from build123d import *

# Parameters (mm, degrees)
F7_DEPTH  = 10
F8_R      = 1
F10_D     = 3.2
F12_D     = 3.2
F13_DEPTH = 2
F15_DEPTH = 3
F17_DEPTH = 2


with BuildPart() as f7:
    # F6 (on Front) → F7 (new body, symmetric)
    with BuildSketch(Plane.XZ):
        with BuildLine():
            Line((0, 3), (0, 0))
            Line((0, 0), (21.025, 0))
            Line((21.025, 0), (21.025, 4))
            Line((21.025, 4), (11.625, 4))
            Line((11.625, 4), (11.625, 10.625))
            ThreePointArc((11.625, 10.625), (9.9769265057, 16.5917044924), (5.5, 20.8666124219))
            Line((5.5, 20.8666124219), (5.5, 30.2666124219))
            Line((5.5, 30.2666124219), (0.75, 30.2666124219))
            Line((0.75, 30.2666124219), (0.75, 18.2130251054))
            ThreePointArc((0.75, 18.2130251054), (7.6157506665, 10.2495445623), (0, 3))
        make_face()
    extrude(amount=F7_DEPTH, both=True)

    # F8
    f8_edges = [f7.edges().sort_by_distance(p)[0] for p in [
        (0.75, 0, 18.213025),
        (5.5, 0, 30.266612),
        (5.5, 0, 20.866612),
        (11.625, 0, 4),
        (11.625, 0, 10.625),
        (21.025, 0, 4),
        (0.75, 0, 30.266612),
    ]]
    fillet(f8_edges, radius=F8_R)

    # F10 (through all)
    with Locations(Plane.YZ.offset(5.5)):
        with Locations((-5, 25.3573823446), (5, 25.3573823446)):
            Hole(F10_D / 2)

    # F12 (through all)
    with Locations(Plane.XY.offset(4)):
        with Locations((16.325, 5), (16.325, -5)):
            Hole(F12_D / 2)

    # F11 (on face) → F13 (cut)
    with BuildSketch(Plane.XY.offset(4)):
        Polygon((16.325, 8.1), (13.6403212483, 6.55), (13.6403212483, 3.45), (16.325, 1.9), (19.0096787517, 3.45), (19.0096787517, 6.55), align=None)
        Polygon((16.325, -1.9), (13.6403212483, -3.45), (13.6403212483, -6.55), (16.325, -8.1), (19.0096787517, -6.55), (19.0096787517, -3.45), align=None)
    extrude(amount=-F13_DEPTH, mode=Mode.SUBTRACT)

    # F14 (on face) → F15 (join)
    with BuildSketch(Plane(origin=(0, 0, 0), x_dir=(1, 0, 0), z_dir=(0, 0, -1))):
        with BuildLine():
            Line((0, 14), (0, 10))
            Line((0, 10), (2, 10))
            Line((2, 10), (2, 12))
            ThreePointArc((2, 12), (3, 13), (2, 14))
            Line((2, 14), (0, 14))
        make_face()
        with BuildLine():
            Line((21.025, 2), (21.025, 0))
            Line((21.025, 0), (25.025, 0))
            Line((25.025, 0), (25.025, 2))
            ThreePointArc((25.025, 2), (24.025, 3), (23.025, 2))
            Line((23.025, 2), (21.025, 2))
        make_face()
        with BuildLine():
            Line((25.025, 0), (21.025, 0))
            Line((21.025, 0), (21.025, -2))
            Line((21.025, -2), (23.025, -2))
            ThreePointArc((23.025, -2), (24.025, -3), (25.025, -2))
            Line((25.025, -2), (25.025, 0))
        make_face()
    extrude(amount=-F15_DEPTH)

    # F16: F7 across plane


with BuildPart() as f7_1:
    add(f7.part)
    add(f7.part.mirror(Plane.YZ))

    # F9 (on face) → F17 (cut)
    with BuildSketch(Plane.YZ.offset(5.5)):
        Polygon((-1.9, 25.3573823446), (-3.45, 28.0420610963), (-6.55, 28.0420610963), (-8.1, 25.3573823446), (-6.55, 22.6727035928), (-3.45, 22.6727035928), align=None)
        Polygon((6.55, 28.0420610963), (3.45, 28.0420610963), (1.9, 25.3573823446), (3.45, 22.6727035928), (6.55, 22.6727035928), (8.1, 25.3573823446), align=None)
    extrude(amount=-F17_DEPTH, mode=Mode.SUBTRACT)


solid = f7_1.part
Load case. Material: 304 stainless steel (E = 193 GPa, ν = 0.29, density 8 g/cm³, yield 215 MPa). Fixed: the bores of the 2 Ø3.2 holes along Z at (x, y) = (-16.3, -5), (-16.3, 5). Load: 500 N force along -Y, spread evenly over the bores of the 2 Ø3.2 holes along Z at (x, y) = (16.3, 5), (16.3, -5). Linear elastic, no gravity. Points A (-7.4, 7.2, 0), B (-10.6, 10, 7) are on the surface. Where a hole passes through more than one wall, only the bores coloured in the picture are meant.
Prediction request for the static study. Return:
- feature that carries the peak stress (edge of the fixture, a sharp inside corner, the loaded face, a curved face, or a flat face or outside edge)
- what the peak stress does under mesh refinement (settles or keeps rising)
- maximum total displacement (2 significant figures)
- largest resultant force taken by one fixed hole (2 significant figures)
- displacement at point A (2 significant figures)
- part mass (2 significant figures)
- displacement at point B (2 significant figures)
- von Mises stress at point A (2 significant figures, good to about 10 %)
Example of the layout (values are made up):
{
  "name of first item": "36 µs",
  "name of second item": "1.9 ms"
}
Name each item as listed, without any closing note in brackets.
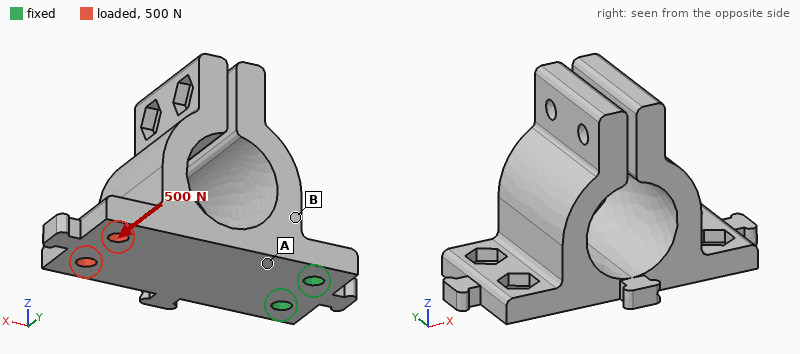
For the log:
{
  "feature that carries the peak stress": "edge of the fixture",
  "what the peak stress does under mesh refinement": "keeps rising",
  "maximum total displacement": "30 µm",
  "largest resultant force taken by one fixed hole": "1.4 kN",
  "displacement at point A": "5.6 µm",
  "part mass": "66 g",
  "displacement at point B": "5.7 µm",
  "von Mises stress at point A": "44 MPa"
}
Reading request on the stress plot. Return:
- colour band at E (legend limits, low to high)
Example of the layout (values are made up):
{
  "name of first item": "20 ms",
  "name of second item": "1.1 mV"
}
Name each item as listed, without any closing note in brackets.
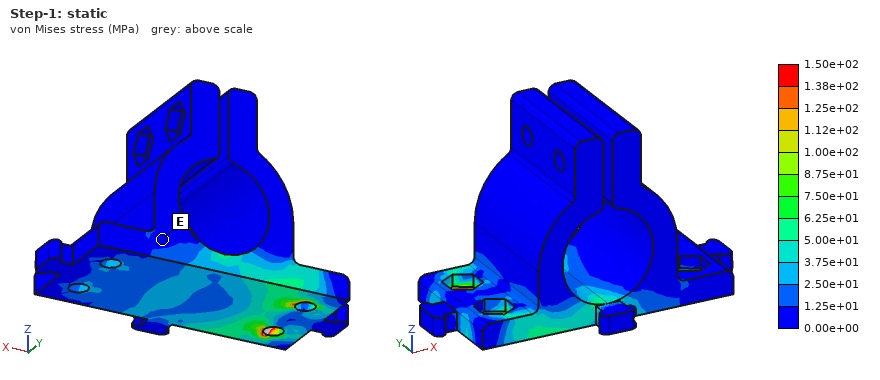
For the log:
{
  "colour band at E": "0.00e+00 to 1.25e+01 MPa"
}
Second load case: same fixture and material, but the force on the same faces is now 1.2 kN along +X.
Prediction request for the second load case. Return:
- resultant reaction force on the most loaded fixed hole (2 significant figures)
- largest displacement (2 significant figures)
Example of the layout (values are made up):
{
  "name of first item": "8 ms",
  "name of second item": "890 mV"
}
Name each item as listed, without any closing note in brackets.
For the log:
{
  "resultant reaction force on the most loaded fixed hole": "600 N",
  "largest displacement": "37 µm"
}
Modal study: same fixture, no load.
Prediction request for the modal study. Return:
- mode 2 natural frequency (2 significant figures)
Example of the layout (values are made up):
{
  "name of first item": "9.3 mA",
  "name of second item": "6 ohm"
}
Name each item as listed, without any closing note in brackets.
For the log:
{
  "mode 2 natural frequency": "2700 Hz"
}
